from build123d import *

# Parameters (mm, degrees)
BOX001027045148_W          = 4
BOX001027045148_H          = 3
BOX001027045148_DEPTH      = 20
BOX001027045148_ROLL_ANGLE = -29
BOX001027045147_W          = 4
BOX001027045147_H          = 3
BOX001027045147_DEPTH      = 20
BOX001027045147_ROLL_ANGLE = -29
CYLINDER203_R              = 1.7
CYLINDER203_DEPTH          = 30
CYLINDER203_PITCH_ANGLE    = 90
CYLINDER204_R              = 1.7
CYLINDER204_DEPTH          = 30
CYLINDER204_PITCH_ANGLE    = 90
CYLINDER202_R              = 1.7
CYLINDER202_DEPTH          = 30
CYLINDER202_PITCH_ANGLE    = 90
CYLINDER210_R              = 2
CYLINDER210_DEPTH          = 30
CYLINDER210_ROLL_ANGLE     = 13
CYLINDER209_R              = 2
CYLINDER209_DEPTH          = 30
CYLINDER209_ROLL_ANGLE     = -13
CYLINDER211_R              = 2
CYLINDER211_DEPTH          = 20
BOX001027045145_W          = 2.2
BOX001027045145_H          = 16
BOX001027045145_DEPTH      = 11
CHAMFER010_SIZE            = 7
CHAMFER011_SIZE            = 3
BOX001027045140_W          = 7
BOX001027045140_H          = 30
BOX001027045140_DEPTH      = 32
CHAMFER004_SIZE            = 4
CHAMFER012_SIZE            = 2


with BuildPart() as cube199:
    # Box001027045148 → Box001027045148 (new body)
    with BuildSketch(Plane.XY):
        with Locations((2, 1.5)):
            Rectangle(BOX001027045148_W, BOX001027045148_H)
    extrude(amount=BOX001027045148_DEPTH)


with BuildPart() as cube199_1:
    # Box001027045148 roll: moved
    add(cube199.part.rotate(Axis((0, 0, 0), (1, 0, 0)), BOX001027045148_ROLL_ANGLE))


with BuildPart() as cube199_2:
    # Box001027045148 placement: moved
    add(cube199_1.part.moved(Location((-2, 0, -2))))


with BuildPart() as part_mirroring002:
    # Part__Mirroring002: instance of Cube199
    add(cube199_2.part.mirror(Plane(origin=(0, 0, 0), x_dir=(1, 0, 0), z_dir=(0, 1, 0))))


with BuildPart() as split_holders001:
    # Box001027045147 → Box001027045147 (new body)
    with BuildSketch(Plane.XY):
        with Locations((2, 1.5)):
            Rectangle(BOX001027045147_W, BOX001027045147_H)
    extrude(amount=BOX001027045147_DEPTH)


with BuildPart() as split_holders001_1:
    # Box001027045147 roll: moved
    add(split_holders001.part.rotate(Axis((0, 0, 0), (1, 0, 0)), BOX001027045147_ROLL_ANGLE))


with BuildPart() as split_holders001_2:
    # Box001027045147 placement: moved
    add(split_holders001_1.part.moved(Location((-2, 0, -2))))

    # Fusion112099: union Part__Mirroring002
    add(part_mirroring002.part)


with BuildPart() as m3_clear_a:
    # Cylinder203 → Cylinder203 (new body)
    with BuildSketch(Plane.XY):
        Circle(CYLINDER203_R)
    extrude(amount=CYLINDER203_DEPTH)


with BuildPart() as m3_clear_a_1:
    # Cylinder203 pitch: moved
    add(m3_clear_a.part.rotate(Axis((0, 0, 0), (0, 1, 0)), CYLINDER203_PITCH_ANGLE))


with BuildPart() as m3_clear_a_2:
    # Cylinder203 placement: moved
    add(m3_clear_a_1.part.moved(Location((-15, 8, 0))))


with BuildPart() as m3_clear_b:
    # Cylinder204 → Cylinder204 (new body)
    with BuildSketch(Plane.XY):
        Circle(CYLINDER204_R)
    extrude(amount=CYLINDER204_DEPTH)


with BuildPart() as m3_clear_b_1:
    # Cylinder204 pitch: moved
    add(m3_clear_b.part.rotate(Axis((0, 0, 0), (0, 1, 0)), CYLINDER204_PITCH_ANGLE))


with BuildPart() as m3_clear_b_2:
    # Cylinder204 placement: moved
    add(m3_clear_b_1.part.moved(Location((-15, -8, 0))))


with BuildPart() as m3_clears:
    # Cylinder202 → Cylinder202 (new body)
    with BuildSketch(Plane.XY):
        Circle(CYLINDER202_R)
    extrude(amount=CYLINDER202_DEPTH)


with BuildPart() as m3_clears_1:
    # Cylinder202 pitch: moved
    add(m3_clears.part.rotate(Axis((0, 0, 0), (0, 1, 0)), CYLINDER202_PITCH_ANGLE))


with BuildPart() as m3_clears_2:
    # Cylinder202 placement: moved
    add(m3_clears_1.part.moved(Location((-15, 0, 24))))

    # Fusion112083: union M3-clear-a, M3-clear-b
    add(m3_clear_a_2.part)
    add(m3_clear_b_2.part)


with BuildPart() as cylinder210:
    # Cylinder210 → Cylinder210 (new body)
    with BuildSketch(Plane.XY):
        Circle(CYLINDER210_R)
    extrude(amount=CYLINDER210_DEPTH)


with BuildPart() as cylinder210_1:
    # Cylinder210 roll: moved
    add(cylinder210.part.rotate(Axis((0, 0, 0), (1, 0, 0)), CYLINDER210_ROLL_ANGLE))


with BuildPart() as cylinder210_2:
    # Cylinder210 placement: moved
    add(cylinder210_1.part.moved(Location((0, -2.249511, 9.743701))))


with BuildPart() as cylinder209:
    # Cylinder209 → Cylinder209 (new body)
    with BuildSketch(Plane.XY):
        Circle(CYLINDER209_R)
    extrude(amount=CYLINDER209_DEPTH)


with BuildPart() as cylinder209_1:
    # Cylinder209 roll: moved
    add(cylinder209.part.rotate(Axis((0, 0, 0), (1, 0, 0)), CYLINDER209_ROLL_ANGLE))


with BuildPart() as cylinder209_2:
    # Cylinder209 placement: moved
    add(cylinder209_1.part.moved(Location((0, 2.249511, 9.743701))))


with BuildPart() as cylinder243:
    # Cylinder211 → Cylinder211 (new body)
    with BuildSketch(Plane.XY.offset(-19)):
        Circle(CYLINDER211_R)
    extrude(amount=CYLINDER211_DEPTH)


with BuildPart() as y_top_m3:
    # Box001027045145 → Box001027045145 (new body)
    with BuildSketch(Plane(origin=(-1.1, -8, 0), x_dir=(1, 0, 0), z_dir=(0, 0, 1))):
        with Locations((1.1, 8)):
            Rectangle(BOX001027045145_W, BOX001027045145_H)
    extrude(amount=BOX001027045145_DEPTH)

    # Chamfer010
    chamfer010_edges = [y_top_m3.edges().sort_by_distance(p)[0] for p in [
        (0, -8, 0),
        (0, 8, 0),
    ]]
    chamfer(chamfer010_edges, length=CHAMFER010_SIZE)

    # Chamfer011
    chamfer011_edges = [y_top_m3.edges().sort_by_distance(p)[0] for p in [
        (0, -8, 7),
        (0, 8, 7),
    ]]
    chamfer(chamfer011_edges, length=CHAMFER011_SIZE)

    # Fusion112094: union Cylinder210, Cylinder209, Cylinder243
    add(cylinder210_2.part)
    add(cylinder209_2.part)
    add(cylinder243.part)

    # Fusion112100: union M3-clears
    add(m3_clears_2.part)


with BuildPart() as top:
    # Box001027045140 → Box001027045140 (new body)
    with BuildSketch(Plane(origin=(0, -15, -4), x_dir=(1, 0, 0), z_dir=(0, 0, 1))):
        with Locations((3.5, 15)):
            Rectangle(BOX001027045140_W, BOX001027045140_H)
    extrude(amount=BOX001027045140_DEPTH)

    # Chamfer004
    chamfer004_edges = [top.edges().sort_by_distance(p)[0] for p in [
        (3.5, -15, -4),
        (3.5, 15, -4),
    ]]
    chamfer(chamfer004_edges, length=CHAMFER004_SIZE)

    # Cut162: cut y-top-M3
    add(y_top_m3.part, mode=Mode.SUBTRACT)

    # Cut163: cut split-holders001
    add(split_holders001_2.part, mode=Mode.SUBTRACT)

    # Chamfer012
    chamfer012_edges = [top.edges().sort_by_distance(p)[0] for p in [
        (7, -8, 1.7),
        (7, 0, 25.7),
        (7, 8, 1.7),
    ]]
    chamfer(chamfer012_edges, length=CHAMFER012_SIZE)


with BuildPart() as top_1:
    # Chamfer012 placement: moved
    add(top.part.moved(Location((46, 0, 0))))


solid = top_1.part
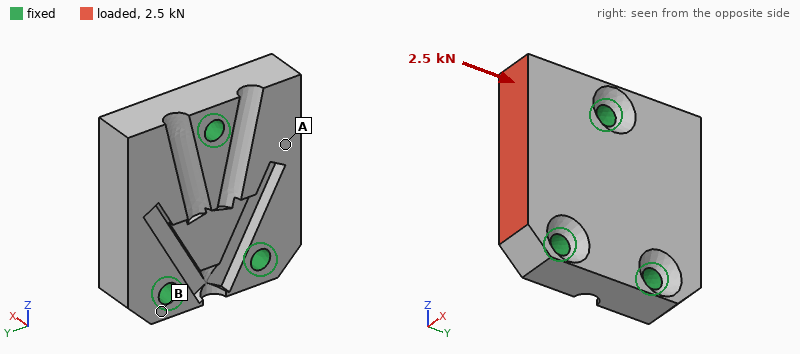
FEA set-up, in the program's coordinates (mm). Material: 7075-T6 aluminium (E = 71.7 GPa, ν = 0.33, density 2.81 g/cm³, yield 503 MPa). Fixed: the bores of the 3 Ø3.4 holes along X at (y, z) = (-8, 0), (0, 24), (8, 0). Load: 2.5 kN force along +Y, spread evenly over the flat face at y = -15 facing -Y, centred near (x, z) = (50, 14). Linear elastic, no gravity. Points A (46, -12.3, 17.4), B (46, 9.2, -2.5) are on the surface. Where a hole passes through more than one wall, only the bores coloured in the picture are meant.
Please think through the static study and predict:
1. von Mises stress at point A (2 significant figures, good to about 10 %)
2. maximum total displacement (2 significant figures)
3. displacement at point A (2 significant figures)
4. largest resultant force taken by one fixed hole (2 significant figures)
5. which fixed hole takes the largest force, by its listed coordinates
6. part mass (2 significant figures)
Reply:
14 MPa
5.9 µm
5.0 µm
1.4 kN
(0, 24)
16 g
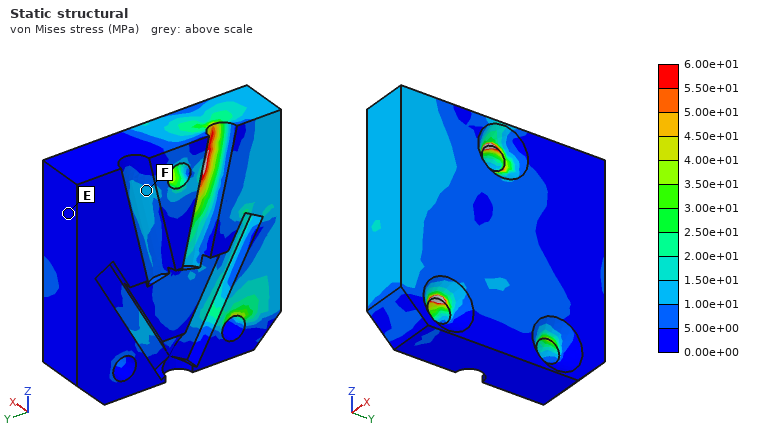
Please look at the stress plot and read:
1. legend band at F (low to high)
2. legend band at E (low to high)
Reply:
1.00e+01 to 1.50e+01 MPa
0.00e+00 to 5.00e+00 MPa
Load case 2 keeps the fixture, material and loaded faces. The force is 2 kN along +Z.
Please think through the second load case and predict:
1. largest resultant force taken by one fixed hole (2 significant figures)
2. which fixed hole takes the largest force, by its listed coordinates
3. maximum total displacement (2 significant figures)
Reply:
1.5 kN
(-8, 0)
11 µm
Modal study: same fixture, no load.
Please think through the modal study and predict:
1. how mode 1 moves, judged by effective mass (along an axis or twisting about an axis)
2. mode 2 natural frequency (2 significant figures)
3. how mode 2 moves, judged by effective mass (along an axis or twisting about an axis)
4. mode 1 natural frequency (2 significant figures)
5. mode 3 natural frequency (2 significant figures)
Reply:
twisting about Z
21 kHz
along X
18 kHz
36 kHz
